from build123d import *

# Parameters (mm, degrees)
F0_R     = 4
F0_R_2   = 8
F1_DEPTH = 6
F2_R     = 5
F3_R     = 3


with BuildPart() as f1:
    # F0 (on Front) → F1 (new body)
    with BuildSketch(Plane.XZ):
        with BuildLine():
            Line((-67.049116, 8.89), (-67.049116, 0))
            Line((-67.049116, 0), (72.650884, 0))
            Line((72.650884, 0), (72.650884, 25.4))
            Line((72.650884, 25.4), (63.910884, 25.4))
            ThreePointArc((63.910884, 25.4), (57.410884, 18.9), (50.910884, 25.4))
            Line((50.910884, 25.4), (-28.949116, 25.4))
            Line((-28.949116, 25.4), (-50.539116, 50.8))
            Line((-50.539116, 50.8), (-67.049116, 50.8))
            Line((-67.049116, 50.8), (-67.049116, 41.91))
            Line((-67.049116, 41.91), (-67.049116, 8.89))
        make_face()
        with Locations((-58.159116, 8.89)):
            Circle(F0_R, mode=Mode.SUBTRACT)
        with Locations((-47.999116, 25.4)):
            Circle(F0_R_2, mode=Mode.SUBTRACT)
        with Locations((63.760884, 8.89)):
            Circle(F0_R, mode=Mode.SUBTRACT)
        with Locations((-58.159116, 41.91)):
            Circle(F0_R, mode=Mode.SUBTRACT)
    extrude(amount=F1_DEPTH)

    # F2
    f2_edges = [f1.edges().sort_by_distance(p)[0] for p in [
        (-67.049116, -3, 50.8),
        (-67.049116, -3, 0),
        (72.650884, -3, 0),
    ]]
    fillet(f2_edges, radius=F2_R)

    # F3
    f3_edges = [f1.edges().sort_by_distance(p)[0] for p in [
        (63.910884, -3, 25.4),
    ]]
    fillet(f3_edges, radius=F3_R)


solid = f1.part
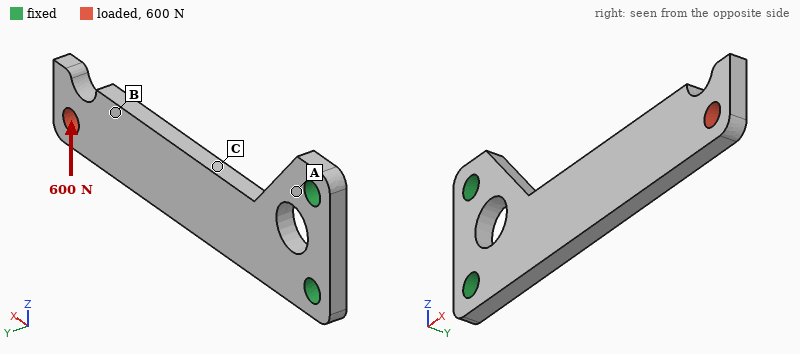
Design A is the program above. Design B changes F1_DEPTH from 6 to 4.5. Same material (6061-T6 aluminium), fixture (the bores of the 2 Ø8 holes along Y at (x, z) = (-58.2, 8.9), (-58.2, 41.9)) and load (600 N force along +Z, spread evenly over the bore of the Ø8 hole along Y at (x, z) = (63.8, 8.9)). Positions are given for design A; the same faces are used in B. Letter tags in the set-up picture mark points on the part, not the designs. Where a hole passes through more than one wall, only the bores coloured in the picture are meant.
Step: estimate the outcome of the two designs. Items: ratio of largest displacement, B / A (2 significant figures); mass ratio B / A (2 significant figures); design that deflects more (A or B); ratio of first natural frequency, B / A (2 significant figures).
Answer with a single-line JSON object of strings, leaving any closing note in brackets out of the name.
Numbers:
{"ratio of largest displacement, B / A": "1.3", "mass ratio B / A": "0.75", "design that deflects more": "B", "ratio of first natural frequency, B / A": "0.76"}
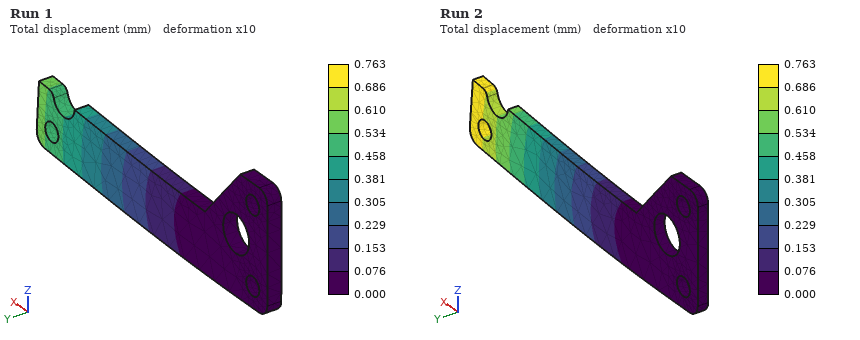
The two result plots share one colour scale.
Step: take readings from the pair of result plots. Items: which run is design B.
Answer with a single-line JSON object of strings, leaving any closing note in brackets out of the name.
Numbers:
{"which run is design B": "Run 2"}
